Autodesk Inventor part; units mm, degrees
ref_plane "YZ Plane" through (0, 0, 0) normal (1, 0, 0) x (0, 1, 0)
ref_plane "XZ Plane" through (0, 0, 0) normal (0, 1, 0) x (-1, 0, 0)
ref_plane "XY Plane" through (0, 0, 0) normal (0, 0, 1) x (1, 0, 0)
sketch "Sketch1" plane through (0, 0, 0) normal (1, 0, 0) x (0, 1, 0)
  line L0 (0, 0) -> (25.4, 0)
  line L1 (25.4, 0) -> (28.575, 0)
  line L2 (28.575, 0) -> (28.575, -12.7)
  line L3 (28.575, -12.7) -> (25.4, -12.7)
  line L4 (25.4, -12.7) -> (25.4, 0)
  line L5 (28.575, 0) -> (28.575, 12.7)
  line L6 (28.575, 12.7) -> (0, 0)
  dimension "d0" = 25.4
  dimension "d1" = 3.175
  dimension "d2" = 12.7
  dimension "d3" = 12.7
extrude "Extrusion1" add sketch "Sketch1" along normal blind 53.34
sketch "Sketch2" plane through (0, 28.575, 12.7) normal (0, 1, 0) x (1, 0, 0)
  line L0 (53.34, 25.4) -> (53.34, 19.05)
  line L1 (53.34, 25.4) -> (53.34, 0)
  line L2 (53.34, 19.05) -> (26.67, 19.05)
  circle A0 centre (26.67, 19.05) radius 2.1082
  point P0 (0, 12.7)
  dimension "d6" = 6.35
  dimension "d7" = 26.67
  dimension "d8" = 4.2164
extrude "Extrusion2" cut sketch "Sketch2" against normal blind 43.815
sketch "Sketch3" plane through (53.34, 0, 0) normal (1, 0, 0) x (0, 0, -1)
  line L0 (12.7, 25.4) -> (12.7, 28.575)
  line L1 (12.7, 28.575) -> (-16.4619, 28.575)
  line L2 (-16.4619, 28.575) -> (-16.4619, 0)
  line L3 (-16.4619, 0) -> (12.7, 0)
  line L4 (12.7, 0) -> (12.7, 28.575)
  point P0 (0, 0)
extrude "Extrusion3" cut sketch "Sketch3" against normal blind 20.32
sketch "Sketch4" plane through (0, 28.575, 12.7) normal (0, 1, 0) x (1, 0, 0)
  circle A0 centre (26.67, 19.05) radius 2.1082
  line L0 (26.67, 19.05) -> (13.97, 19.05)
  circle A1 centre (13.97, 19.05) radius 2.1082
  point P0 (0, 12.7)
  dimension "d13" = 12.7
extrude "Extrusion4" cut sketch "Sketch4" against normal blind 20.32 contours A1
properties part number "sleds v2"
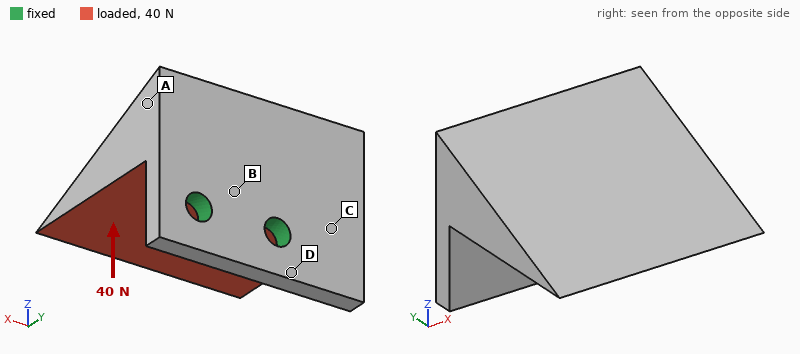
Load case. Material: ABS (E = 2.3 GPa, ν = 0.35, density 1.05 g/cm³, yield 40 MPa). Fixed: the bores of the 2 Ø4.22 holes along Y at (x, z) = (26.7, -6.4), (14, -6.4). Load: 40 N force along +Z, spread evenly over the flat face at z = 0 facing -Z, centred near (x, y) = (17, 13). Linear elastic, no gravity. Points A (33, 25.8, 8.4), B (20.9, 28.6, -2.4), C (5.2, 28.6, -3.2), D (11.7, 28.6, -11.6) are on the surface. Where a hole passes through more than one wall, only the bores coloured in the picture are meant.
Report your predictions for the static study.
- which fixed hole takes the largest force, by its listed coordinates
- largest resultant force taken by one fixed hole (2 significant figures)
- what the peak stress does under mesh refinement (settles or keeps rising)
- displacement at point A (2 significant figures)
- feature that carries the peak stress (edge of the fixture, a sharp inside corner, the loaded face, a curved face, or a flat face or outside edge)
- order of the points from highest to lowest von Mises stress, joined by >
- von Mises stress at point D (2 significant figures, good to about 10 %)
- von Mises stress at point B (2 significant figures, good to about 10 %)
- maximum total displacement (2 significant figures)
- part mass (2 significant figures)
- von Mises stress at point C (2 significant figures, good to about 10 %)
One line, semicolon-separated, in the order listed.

(14, -6.4); 30 N; keeps rising; 0.21 mm; edge of the fixture; B > C > D > A; 3.0 MPa; 8.3 MPa; 0.60 mm; 7.6 g; 5.8 MPa
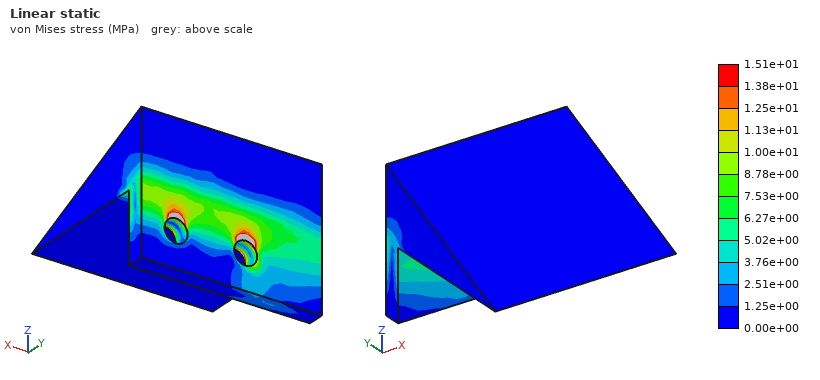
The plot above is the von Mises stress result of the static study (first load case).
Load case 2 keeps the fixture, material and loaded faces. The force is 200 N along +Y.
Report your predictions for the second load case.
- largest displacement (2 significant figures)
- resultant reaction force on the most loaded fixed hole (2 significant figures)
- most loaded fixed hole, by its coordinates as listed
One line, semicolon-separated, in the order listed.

0.42 mm; 140 N; (14, -6.4)
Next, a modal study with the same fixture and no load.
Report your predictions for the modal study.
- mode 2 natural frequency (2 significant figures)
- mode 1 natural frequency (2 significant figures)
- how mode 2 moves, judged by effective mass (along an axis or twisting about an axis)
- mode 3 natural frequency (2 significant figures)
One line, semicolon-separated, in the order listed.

1800 Hz; 830 Hz; along X; 3700 Hz
